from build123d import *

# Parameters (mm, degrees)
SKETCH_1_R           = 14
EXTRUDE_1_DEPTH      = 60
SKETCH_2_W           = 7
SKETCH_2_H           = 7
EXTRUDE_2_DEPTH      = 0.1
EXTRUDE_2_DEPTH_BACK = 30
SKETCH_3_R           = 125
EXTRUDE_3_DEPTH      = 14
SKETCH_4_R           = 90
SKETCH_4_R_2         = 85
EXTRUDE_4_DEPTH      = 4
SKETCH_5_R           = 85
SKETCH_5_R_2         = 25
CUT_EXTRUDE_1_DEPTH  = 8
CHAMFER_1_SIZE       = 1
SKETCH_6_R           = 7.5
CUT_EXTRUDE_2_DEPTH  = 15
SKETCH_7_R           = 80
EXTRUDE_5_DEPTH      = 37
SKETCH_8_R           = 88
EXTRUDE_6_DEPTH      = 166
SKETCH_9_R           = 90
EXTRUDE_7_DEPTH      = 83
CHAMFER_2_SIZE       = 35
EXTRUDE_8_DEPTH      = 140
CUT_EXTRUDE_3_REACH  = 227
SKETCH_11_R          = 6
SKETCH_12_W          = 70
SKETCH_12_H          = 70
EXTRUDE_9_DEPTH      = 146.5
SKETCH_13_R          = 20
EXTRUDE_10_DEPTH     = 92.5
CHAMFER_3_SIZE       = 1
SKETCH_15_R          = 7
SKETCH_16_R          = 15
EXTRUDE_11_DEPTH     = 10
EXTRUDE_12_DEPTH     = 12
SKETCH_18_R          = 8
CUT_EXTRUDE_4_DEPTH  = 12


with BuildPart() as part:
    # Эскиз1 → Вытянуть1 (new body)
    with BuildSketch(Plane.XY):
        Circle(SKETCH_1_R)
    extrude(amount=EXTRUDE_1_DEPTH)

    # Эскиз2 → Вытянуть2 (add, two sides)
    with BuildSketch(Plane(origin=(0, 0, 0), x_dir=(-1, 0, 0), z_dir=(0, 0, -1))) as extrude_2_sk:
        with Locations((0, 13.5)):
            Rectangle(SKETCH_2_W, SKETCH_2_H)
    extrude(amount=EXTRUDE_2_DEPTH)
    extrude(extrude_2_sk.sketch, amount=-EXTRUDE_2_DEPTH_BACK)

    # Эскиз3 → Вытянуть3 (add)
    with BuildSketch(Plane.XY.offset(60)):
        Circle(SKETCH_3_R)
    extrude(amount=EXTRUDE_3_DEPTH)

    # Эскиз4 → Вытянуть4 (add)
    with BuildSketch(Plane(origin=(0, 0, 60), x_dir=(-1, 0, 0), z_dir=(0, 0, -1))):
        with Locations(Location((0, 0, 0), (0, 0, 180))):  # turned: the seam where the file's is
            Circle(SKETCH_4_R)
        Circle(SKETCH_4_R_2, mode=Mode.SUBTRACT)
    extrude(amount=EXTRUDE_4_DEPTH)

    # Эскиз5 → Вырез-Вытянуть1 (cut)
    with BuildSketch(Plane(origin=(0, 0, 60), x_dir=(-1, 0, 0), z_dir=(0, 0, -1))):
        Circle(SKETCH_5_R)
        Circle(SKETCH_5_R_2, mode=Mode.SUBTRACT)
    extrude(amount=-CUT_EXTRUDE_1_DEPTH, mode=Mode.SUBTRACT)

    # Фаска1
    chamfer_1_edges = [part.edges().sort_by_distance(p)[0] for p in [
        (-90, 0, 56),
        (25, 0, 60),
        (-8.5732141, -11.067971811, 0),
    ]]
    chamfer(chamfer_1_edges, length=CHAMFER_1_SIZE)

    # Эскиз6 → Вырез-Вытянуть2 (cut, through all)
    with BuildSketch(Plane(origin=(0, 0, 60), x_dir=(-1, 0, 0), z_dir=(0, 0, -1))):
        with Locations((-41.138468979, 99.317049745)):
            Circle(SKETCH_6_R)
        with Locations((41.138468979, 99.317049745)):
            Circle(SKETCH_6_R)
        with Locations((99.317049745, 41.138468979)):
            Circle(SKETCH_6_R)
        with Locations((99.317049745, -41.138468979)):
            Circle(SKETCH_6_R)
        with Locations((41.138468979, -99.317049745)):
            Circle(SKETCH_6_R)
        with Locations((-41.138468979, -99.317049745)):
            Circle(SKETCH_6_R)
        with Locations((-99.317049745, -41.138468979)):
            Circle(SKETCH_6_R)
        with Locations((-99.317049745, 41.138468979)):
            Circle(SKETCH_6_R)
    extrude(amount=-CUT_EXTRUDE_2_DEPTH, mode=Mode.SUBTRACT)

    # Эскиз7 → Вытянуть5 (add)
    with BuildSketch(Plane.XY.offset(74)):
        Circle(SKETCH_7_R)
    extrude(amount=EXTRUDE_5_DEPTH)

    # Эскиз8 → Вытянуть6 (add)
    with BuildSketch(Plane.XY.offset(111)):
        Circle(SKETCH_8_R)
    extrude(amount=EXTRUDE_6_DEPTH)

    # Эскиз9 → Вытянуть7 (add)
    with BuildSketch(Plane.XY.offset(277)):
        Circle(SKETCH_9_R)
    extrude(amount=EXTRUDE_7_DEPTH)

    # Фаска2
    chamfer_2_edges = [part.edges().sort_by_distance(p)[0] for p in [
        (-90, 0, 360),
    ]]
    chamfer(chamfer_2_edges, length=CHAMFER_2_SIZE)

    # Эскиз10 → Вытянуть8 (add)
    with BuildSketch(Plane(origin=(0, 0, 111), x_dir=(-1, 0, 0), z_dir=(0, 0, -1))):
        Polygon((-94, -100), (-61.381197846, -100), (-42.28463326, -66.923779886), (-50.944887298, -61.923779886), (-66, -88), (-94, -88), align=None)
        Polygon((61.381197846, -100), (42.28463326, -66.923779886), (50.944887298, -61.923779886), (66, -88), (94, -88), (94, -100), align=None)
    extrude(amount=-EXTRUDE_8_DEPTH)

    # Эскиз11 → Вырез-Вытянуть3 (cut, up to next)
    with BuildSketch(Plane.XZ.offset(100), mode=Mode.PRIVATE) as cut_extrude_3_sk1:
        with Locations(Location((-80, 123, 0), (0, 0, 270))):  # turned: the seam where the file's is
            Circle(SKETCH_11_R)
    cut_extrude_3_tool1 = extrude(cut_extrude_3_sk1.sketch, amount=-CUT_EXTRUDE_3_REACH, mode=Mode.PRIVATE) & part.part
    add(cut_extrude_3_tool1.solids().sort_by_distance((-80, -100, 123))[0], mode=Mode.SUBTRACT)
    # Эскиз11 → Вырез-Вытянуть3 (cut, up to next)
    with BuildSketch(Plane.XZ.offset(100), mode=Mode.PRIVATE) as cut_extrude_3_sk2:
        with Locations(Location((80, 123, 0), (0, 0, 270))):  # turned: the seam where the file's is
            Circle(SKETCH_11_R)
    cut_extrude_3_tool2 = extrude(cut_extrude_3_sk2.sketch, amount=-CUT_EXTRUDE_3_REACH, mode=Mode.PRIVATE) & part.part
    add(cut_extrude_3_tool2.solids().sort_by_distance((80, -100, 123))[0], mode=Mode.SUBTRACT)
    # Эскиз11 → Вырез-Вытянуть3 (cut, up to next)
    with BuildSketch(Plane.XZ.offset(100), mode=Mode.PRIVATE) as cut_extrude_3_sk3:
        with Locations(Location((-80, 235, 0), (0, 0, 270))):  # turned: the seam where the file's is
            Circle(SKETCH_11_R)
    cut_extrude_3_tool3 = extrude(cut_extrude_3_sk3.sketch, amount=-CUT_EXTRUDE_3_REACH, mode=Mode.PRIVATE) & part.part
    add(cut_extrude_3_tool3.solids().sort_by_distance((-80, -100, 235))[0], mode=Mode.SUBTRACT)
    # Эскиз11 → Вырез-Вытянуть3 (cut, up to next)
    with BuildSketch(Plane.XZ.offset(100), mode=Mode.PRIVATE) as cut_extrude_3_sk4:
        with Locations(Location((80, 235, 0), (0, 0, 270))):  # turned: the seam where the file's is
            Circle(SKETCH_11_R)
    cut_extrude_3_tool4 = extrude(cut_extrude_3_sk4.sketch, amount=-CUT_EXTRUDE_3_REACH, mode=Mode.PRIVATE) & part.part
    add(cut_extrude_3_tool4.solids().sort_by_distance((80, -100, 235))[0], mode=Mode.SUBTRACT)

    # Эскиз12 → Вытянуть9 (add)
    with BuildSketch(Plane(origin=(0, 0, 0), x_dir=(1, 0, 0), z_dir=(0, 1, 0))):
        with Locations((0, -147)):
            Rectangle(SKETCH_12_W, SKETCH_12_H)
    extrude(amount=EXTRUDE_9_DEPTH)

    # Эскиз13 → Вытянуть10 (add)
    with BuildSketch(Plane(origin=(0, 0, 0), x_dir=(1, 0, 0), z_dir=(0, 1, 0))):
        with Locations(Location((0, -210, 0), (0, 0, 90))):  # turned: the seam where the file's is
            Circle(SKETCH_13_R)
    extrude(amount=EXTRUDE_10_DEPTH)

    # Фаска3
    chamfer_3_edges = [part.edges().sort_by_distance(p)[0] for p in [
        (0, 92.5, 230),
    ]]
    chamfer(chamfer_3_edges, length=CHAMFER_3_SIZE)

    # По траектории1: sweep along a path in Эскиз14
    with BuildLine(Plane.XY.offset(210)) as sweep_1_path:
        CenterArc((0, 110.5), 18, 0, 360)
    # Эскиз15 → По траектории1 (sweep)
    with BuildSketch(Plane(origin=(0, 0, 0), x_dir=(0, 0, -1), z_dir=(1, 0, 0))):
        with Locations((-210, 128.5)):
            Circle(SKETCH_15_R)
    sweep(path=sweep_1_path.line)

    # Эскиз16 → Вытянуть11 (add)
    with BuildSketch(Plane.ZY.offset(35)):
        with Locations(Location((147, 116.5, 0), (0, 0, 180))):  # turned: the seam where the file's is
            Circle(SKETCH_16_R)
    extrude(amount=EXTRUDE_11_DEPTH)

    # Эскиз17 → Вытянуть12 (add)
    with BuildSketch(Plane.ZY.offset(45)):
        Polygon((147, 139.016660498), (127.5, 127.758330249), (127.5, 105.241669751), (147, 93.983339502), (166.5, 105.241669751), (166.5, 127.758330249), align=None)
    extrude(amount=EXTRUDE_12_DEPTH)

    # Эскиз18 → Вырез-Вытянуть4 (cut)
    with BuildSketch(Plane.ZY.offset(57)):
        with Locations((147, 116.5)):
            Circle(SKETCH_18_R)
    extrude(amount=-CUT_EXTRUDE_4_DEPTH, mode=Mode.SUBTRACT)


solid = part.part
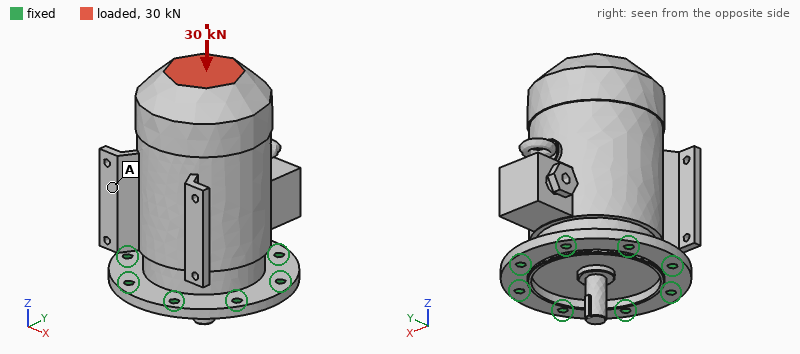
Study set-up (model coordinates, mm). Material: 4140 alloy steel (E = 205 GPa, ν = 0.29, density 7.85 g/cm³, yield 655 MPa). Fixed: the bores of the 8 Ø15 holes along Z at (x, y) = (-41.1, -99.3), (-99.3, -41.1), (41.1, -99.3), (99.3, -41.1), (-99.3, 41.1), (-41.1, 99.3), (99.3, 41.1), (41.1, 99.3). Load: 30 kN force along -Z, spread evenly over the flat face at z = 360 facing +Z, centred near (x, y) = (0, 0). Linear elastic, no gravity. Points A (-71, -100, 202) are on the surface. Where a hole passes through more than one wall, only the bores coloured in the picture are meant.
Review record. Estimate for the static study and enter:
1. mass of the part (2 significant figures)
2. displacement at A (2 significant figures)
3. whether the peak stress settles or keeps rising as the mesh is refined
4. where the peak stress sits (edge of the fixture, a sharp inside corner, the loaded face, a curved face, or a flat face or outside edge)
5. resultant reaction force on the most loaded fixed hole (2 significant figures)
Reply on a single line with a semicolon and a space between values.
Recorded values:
60 kg; 8.7 µm; keeps rising; edge of the fixture; 5.0 kN
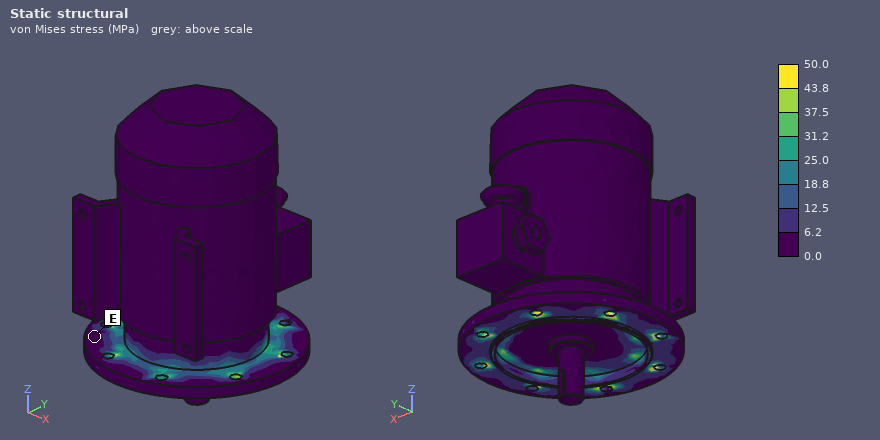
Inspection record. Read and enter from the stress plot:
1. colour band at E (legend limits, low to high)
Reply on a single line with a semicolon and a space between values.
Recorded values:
0.0 to 6.2 MPa
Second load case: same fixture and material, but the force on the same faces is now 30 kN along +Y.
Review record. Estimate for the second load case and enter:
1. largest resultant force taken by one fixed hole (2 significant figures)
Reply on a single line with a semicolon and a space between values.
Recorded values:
26 kN
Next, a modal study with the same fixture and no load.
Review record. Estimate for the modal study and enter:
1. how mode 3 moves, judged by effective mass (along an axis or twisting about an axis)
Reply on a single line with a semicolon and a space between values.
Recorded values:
along Z
